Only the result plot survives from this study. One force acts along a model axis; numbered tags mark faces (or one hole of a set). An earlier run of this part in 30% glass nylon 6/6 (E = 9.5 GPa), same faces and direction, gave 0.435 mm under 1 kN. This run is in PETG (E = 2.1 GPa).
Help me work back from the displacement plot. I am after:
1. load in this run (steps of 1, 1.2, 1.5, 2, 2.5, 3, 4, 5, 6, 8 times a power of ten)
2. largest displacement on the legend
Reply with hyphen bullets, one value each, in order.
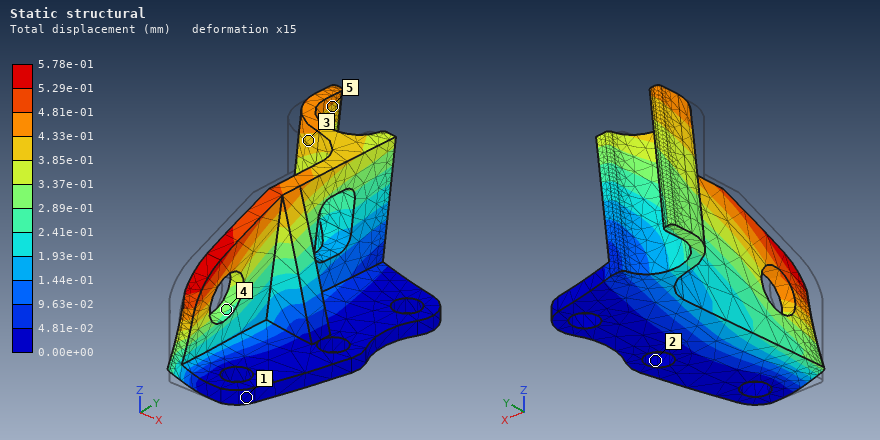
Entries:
- 300 N
- 5.78e-01 mm
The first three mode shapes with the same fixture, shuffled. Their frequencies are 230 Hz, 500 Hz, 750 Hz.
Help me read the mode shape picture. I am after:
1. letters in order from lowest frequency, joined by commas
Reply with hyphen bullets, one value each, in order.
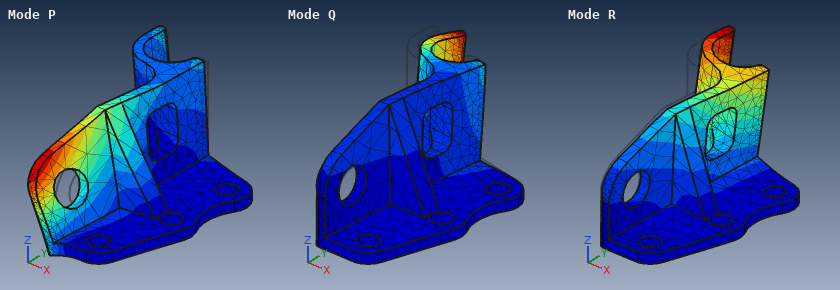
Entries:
- R, Q, P
